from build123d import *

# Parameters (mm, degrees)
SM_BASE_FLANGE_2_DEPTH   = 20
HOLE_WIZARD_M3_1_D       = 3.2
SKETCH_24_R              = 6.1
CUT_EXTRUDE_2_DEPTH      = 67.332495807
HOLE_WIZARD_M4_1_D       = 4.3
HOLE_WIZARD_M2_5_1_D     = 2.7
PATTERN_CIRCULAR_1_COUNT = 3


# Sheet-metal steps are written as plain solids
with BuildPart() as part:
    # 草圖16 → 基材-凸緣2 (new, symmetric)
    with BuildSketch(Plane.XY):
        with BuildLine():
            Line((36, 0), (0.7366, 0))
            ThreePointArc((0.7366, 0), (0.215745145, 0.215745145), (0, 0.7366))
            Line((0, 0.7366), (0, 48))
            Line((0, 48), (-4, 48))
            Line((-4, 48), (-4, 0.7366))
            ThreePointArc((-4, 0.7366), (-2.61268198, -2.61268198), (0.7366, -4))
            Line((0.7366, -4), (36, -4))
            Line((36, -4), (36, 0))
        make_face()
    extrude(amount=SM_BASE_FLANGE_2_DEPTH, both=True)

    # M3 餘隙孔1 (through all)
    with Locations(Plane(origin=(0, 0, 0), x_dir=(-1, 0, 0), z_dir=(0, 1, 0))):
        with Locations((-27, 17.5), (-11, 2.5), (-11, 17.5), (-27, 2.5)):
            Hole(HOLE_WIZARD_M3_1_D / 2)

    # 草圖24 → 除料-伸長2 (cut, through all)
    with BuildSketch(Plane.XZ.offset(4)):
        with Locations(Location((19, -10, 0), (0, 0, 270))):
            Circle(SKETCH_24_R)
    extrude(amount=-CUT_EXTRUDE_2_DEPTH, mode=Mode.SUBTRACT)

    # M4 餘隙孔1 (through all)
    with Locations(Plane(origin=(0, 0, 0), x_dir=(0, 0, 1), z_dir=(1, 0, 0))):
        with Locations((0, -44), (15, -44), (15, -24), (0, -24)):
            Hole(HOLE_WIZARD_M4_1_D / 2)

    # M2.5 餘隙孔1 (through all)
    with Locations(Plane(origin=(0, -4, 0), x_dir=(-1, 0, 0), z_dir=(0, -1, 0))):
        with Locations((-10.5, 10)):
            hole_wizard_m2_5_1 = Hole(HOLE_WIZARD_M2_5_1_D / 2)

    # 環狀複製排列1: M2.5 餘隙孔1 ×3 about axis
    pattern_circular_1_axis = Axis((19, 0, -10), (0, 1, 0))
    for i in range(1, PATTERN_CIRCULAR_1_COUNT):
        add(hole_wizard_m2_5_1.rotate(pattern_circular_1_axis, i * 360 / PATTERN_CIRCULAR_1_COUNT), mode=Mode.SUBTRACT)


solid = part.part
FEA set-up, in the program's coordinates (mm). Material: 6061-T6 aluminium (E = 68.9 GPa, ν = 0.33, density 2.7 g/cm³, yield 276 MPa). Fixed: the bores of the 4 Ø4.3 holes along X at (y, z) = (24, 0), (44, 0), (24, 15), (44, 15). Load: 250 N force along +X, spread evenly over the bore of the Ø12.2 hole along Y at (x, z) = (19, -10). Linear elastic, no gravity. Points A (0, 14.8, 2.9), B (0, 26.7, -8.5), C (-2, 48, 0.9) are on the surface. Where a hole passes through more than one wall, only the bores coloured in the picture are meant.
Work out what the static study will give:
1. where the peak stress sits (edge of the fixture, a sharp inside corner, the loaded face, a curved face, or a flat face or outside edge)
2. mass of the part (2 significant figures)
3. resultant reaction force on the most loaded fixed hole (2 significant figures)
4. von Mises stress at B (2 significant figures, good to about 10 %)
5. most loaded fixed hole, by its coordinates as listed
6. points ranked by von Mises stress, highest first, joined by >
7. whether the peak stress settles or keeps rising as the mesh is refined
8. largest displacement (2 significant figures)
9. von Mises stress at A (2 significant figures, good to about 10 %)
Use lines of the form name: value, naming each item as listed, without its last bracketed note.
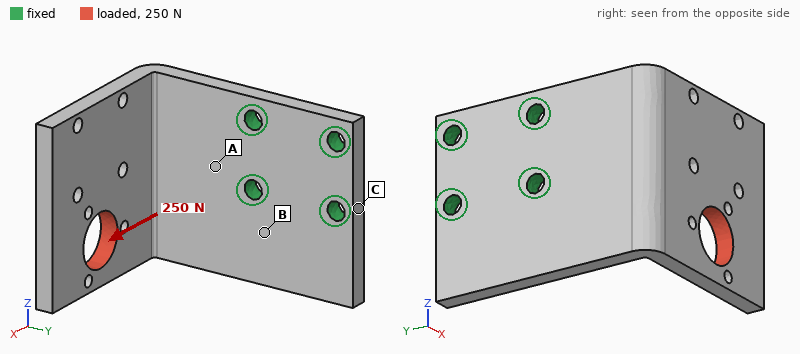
where the peak stress sits: edge of the fixture
mass of the part: 35 g
resultant reaction force on the most loaded fixed hole: 410 N
von Mises stress at B: 33 MPa
most loaded fixed hole, by its coordinates as listed: (24, 0)
points ranked by von Mises stress, highest first, joined by >: A > B > C
whether the peak stress settles or keeps rising as the mesh is refined: keeps rising
largest displacement: 0.31 mm
von Mises stress at A: 45 MPa
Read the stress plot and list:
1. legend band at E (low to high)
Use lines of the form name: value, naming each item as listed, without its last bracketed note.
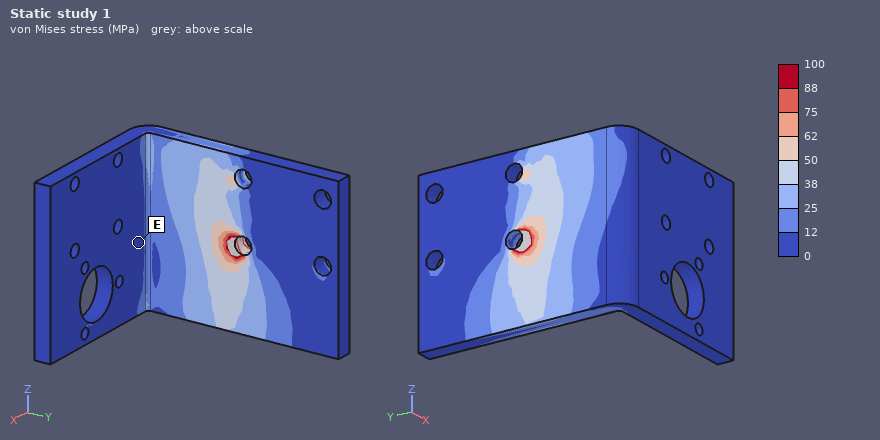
legend band at E: 0 to 12 MPa
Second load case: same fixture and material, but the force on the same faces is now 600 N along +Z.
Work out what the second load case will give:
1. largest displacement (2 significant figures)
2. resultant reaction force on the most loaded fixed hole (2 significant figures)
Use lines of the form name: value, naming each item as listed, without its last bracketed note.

largest displacement: 0.46 mm
resultant reaction force on the most loaded fixed hole: 950 N
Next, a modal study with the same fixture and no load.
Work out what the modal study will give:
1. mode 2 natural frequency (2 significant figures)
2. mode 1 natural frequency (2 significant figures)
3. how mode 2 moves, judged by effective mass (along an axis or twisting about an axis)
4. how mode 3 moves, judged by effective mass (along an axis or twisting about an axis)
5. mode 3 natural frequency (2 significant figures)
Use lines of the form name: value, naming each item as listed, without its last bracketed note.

mode 2 natural frequency: 1800 Hz
mode 1 natural frequency: 1100 Hz
how mode 2 moves, judged by effective mass: along Z
how mode 3 moves, judged by effective mass: along X
mode 3 natural frequency: 3100 Hz
